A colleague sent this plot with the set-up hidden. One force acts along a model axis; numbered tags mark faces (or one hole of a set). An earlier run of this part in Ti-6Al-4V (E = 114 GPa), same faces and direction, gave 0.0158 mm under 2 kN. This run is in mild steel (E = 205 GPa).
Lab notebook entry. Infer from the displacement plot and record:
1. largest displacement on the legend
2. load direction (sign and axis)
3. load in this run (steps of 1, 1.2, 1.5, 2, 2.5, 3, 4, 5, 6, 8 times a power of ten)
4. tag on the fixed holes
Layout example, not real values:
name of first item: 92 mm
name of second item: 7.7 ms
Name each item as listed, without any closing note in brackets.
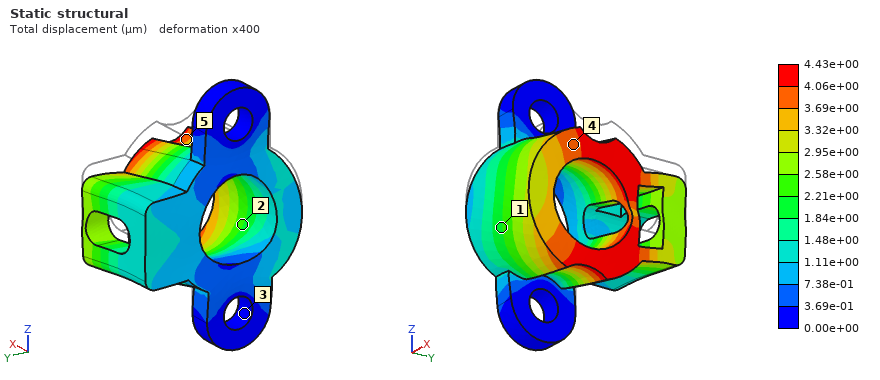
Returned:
largest displacement on the legend: 4.43e+00 µm
load direction: -Z
load in this run: 1 kN
tag on the fixed holes: 3
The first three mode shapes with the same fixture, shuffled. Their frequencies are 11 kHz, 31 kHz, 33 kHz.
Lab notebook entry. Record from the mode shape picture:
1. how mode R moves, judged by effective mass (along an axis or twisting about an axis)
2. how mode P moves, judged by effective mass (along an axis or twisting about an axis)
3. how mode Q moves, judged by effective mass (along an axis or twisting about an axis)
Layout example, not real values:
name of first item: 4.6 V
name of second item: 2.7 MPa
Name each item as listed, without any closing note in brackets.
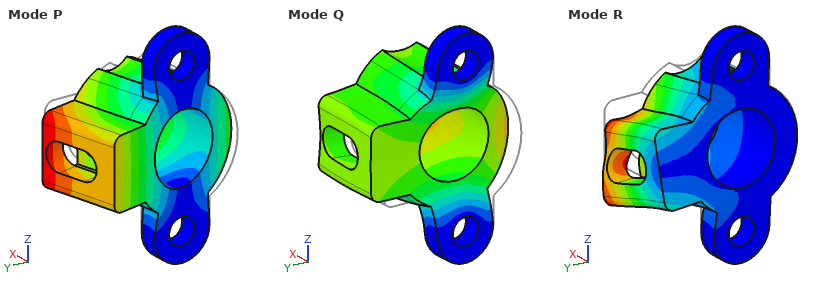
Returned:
how mode R moves, judged by effective mass: along Z
how mode P moves, judged by effective mass: along Y
how mode Q moves, judged by effective mass: along X
